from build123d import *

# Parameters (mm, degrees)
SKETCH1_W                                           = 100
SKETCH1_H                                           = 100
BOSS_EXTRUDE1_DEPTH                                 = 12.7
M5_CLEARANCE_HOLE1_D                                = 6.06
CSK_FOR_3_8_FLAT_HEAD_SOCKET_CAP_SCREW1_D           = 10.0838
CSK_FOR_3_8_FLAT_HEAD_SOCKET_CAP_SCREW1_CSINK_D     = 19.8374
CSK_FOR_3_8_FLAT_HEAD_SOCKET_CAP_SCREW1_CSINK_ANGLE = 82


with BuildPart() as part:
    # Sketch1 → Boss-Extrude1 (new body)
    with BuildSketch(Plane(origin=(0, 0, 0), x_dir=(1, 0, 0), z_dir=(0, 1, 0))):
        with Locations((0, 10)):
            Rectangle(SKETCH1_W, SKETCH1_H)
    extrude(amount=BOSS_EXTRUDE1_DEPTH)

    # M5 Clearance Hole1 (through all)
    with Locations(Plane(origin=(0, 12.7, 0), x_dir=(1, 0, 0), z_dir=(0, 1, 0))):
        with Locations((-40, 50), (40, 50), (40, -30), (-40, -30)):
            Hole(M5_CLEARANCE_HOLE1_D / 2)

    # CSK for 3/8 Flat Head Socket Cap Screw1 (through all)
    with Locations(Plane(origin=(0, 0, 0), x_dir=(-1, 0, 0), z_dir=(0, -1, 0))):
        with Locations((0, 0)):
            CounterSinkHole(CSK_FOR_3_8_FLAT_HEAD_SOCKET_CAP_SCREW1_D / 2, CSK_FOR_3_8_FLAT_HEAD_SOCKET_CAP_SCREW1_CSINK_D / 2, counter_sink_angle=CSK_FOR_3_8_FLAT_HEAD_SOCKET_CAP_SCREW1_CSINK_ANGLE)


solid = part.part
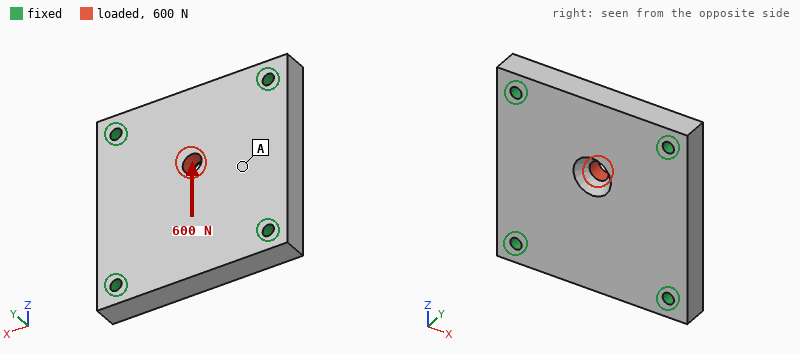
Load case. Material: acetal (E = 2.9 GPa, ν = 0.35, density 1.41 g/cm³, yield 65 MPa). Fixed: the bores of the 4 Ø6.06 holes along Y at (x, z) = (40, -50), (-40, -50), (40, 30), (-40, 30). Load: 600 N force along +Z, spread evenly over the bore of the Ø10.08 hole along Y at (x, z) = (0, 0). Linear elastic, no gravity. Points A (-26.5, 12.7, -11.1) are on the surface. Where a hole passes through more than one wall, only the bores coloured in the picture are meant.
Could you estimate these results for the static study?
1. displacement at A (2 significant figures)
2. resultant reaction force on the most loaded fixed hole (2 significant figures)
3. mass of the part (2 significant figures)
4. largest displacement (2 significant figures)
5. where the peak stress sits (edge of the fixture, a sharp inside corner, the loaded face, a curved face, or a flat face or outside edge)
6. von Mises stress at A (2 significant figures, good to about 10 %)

6.7 µm
180 N
170 g
22 µm
the loaded face
0.52 MPa
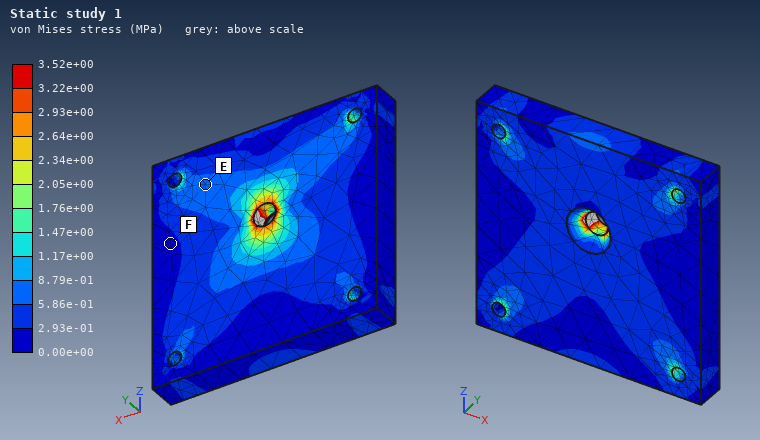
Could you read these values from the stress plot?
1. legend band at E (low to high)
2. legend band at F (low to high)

5.86e-01 to 8.79e-01 MPa
0.00e+00 to 2.93e-01 MPa
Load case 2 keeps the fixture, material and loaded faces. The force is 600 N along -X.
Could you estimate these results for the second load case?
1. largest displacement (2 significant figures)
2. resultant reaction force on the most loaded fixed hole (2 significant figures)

20 µm
200 N
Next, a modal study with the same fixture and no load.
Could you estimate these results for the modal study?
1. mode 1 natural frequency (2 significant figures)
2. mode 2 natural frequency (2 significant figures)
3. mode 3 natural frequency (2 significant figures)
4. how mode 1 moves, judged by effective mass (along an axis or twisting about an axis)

1700 Hz
2700 Hz
2700 Hz
along Y
